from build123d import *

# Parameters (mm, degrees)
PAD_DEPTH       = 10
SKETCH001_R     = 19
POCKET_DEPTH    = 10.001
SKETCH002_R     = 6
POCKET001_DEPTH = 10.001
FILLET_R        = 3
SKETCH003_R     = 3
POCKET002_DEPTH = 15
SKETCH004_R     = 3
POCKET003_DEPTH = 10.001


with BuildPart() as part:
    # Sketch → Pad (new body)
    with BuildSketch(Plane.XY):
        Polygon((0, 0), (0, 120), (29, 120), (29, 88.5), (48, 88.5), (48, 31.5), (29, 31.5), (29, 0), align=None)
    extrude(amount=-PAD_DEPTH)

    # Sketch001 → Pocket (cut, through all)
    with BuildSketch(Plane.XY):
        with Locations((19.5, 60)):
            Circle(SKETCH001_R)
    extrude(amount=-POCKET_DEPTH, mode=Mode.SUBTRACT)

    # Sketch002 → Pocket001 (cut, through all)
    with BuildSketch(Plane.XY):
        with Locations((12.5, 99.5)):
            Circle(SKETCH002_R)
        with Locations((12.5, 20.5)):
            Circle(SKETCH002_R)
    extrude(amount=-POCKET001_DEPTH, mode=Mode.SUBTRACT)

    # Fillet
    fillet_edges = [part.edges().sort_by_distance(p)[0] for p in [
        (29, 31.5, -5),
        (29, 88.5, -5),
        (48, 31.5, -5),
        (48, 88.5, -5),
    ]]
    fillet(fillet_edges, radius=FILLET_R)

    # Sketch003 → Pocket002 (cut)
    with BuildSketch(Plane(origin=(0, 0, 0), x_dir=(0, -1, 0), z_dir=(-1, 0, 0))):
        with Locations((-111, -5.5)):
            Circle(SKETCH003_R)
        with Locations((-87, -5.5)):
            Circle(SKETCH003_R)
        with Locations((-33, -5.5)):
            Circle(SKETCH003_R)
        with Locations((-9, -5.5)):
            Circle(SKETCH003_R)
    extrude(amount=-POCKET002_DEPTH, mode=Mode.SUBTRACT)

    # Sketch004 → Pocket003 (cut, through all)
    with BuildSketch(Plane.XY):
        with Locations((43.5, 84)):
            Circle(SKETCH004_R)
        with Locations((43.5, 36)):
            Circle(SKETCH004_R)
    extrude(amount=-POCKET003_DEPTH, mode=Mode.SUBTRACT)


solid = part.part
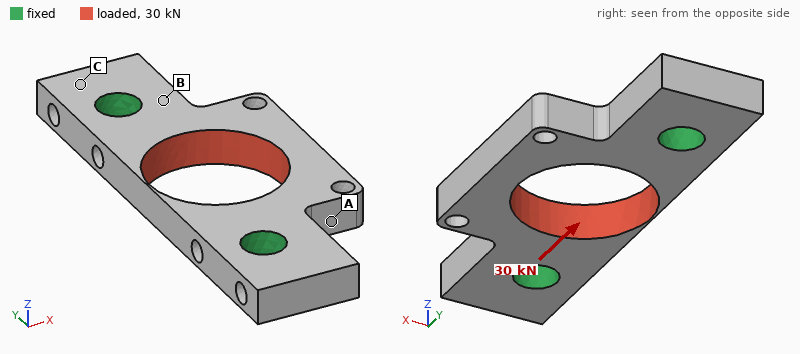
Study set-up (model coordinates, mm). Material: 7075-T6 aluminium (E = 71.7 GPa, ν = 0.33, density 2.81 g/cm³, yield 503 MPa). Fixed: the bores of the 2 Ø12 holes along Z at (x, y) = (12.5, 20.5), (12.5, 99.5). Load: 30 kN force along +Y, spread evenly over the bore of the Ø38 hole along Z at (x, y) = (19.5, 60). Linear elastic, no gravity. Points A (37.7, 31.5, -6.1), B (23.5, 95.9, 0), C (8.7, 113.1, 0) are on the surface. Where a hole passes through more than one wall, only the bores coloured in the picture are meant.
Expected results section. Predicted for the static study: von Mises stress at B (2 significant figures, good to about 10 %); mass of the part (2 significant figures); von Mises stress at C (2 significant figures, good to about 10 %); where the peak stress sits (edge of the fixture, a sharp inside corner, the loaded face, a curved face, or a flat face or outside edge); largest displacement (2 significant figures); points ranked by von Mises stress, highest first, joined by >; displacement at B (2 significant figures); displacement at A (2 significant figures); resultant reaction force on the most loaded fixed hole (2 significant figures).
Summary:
64 MPa
84 g
18 MPa
a curved face
68 µm
B > A > C
12 µm
52 µm
15 kN
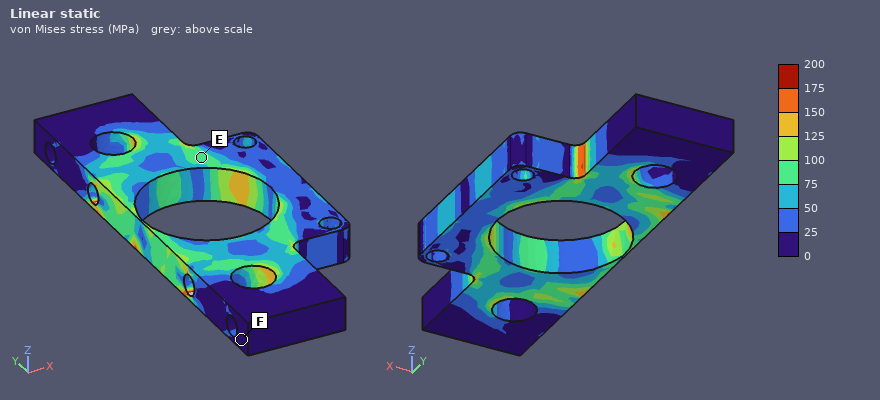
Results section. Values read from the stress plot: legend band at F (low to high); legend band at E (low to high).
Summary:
0 to 25 MPa
75 to 100 MPa
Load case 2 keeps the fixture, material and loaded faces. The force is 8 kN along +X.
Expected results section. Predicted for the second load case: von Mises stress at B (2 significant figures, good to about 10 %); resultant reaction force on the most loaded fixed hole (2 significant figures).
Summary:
16 MPa
4.0 kN
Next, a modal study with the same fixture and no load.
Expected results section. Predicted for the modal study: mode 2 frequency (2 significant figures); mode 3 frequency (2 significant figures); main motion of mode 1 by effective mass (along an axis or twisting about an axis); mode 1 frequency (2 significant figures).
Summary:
10 kHz
13 kHz
along Z
4800 Hz
